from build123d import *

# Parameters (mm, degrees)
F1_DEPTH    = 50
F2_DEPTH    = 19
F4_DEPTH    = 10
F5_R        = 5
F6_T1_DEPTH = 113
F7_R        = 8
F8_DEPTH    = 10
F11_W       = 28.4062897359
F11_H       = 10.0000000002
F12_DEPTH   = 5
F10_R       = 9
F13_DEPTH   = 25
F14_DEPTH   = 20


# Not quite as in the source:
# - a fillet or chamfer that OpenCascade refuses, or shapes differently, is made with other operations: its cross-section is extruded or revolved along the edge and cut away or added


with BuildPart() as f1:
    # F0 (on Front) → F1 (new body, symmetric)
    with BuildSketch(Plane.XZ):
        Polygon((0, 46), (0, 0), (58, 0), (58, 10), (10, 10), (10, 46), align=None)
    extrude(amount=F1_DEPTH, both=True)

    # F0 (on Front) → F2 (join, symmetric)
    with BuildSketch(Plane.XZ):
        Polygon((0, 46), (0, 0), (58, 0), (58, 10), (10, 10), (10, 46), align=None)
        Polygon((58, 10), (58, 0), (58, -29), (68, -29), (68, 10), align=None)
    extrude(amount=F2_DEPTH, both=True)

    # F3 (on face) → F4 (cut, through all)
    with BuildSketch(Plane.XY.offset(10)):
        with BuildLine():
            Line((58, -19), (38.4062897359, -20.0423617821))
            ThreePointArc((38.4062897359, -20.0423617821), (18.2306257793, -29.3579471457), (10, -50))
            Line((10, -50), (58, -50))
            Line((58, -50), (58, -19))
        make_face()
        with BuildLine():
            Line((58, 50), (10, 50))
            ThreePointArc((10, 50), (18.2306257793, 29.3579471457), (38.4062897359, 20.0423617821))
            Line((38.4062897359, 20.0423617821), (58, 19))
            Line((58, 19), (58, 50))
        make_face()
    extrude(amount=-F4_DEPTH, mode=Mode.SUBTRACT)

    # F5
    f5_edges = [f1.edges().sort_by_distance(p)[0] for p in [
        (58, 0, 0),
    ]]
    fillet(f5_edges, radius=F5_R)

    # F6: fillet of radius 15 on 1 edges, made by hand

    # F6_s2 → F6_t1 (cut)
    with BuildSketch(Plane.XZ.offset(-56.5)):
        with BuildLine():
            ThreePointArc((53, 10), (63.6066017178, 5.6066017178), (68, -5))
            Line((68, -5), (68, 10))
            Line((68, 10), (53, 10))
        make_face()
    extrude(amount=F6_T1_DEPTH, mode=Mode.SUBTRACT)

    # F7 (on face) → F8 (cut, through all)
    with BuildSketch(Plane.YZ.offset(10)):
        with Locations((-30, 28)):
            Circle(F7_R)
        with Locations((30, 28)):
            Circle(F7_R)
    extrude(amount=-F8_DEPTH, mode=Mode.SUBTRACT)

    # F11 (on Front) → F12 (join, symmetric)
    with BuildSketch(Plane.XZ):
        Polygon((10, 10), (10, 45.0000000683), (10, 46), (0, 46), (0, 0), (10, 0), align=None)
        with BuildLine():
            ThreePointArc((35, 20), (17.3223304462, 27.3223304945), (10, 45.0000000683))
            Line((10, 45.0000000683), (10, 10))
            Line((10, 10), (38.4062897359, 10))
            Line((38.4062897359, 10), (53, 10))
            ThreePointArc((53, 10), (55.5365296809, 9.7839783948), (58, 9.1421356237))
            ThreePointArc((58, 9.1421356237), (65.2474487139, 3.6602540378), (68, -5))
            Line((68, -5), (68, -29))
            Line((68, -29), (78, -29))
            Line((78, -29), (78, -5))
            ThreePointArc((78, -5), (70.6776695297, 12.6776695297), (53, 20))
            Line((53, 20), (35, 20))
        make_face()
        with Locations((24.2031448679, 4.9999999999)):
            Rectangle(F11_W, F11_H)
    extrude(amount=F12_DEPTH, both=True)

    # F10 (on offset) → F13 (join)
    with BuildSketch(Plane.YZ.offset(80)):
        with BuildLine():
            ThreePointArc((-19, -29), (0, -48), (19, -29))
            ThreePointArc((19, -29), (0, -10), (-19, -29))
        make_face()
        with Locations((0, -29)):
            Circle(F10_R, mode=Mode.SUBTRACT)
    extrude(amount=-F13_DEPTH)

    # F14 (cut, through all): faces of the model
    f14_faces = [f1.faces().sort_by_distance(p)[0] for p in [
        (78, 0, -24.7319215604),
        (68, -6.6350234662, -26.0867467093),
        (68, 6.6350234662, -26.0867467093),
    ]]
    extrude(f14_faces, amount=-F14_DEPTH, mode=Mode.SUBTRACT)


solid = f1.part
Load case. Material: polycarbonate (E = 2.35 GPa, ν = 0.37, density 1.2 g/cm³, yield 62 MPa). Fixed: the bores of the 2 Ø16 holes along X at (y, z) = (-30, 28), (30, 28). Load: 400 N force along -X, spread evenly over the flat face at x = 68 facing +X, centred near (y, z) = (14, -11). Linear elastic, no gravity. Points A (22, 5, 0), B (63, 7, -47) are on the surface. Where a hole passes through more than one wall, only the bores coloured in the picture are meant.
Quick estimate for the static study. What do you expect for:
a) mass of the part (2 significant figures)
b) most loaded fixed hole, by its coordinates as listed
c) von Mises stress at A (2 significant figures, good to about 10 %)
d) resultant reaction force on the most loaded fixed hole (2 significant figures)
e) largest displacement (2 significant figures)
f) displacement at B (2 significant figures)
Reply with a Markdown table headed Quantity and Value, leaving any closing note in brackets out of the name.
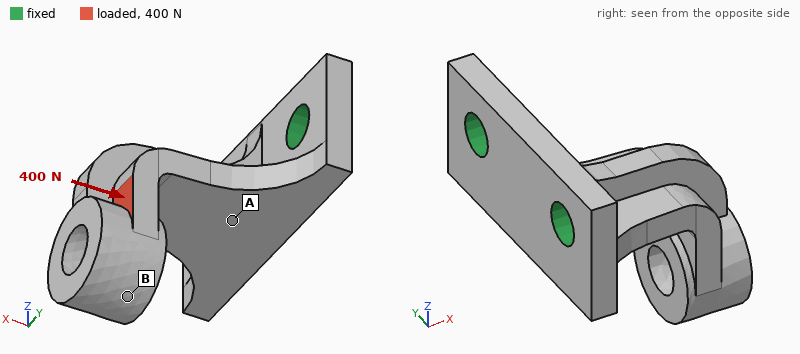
| Quantity | Value |
|---|---|
| mass of the part | 120 g |
| most loaded fixed hole, by its coordinates as listed | (30, 28) |
| von Mises stress at A | 3.0 MPa |
| resultant reaction force on the most loaded fixed hole | 300 N |
| largest displacement | 1.5 mm |
| displacement at B | 1.4 mm |
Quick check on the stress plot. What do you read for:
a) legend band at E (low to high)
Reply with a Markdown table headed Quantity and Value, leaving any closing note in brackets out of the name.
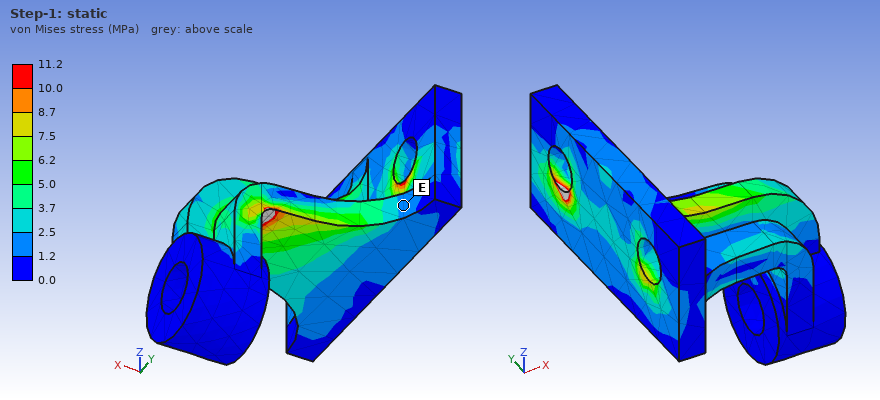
| Quantity | Value |
|---|---|
| legend band at E | 1.2 to 2.5 MPa |
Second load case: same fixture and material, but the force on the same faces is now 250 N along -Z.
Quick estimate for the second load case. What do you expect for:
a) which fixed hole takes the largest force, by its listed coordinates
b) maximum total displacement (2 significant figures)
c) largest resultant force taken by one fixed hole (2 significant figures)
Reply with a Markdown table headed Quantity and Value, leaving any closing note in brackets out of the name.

| Quantity | Value |
|---|---|
| which fixed hole takes the largest force, by its listed coordinates | (30, 28) |
| maximum total displacement | 1.7 mm |
| largest resultant force taken by one fixed hole | 180 N |
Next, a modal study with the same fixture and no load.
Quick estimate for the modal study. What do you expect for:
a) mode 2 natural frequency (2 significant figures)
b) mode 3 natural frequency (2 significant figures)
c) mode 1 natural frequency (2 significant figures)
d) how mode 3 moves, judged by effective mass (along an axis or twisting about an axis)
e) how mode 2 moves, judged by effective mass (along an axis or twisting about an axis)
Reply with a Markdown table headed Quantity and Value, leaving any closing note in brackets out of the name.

| Quantity | Value |
|---|---|
| mode 2 natural frequency | 440 Hz |
| mode 3 natural frequency | 950 Hz |
| mode 1 natural frequency | 320 Hz |
| how mode 3 moves, judged by effective mass | along Z |
| how mode 2 moves, judged by effective mass | along Y |
